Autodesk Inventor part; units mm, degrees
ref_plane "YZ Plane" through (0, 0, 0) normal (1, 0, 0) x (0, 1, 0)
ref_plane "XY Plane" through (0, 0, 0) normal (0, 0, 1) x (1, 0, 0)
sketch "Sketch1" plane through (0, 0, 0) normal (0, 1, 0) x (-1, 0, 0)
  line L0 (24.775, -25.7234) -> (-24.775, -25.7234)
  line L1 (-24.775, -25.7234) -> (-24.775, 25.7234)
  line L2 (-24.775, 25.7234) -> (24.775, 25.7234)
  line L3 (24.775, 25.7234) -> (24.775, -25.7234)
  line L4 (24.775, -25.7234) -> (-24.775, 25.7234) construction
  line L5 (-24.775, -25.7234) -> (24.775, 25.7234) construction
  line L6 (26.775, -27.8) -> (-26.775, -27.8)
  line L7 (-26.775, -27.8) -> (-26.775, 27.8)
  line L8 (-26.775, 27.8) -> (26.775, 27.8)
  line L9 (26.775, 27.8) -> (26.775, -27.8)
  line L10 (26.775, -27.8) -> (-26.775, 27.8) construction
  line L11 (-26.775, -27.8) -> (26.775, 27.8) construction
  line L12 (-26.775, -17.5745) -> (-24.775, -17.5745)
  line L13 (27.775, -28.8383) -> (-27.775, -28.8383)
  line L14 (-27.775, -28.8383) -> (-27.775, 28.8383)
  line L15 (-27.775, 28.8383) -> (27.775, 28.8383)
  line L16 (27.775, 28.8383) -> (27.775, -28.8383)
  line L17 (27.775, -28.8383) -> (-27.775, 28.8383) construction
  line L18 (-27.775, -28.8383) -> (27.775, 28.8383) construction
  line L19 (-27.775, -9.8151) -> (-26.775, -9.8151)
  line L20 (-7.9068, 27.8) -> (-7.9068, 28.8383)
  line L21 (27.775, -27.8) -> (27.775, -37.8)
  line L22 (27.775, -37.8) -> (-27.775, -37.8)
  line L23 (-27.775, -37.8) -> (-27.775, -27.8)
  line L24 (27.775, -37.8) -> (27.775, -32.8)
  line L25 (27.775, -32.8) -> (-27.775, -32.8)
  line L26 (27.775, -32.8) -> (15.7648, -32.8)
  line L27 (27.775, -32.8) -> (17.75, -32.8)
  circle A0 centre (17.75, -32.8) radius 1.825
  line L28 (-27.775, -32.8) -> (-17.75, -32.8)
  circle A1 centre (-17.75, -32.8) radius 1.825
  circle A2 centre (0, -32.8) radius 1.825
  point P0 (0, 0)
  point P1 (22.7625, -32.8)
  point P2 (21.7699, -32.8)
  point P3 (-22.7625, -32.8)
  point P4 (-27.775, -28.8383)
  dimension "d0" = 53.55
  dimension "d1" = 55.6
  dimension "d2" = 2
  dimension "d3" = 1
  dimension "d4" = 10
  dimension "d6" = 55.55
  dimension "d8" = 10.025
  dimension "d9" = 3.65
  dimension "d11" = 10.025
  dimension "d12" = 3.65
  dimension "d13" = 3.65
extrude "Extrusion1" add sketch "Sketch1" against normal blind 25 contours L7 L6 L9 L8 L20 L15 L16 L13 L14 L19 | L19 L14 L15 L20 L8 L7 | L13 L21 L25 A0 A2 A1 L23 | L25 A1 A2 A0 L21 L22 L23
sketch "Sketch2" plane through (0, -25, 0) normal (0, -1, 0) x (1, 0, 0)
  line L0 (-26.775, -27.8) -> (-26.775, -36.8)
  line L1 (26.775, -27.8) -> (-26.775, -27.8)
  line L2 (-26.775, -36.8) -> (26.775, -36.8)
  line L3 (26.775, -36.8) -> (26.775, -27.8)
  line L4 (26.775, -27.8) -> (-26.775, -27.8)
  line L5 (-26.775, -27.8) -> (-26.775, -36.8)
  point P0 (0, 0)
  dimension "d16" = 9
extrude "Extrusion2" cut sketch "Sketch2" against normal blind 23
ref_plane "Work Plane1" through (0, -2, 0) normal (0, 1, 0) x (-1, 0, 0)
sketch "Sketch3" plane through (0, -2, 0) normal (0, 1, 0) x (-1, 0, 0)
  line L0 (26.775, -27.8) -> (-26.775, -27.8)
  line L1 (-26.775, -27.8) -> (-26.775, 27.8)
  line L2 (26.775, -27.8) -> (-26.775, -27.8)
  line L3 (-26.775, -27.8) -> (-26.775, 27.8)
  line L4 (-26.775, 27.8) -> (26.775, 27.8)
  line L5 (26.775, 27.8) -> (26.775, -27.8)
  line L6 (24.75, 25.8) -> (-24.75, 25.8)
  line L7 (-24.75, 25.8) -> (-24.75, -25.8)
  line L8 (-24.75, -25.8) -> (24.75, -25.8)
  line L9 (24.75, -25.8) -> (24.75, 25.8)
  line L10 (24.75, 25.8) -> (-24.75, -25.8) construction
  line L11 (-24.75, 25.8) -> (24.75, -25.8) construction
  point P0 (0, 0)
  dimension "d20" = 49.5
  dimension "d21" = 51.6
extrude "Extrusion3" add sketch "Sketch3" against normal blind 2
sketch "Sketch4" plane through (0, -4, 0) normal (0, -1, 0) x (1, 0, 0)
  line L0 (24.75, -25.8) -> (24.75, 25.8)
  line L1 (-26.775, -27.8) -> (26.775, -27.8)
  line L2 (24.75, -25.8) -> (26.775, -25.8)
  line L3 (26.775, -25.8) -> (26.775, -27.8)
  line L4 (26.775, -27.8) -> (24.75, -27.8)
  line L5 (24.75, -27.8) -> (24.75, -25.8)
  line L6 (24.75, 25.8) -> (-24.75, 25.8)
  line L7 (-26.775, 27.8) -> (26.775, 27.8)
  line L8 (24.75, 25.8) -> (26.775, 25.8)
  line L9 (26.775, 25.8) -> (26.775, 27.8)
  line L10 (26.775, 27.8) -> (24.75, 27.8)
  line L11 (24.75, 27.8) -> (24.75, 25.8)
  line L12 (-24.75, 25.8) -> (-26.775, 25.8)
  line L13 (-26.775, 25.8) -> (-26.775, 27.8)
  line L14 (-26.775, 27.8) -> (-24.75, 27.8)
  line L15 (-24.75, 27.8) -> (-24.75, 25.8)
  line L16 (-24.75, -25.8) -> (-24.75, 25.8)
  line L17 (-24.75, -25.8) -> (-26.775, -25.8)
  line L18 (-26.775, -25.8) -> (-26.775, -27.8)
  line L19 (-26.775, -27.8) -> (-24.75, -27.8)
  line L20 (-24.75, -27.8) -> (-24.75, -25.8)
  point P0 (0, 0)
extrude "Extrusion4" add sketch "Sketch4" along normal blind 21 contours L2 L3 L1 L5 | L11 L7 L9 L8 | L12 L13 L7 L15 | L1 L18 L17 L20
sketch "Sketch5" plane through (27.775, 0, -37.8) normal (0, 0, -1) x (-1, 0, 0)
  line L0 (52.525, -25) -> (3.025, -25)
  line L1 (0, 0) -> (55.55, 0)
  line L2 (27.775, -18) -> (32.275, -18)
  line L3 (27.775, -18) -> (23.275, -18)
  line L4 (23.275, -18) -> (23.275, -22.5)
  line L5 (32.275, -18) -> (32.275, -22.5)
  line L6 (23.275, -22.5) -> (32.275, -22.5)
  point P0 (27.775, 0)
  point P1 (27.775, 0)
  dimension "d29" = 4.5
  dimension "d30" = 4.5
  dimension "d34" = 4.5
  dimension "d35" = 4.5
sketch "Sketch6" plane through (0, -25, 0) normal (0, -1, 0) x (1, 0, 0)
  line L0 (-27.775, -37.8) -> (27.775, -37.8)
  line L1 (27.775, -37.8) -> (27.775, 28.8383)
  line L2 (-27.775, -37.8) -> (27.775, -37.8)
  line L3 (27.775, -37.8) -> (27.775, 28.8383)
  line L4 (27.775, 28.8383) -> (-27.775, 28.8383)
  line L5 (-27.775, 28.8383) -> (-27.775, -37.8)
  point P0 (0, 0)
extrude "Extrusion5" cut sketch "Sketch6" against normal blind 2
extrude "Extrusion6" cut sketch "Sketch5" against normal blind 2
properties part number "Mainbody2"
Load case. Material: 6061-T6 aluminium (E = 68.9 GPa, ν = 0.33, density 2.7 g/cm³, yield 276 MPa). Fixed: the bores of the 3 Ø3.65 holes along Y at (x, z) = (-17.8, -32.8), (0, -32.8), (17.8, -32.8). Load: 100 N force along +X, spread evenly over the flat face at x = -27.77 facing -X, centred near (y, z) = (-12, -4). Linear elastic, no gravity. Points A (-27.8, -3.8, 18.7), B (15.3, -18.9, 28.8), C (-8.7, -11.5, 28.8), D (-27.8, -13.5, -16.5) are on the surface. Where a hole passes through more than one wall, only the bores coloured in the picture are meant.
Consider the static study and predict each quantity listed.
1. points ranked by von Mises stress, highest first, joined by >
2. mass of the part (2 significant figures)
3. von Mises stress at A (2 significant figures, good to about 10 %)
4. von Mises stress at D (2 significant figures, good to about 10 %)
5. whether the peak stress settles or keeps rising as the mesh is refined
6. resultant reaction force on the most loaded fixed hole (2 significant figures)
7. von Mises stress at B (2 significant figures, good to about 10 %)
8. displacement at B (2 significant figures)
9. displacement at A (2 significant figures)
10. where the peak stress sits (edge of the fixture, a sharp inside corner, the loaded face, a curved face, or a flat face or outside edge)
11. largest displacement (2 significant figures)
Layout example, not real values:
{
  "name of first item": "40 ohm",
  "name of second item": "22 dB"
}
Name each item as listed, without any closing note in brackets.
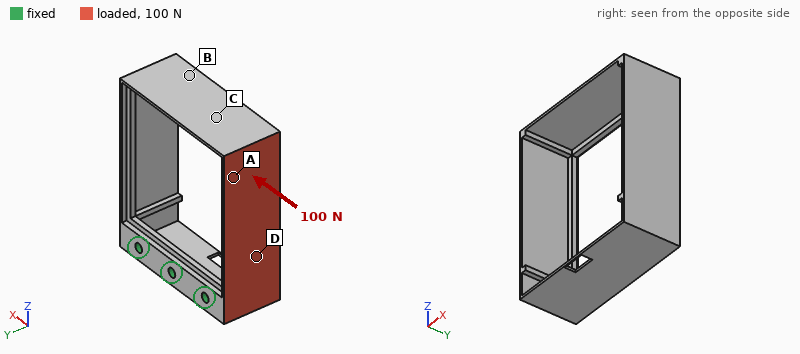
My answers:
{
  "points ranked by von Mises stress, highest first, joined by >": "A > D > B > C",
  "mass of the part": "20 g",
  "von Mises stress at A": "45 MPa",
  "von Mises stress at D": "29 MPa",
  "whether the peak stress settles or keeps rising as the mesh is refined": "keeps rising",
  "resultant reaction force on the most loaded fixed hole": "76 N",
  "von Mises stress at B": "16 MPa",
  "displacement at B": "0.73 mm",
  "displacement at A": "0.63 mm",
  "where the peak stress sits": "a sharp inside corner",
  "largest displacement": "0.80 mm"
}
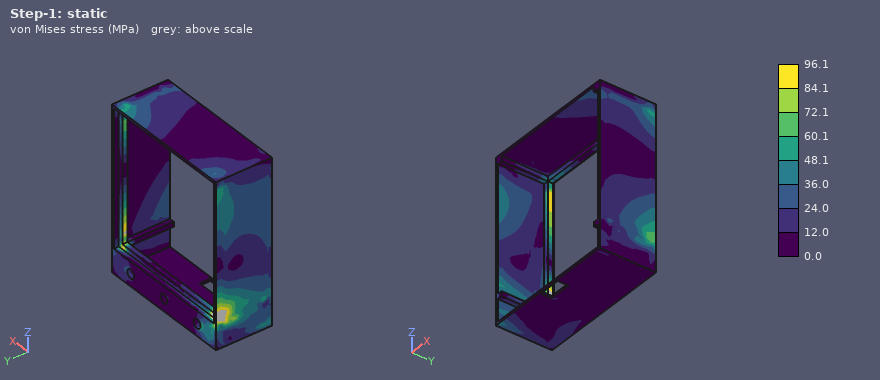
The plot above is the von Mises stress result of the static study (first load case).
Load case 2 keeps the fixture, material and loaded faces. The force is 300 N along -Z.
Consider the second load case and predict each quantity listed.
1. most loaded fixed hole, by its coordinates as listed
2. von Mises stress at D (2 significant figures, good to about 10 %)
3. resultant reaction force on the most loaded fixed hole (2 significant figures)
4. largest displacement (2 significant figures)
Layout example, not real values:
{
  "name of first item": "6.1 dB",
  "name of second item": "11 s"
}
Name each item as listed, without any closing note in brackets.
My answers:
{
  "most loaded fixed hole, by its coordinates as listed": "(-17.8, -32.8)",
  "von Mises stress at D": "20 MPa",
  "resultant reaction force on the most loaded fixed hole": "370 N",
  "largest displacement": "0.94 mm"
}
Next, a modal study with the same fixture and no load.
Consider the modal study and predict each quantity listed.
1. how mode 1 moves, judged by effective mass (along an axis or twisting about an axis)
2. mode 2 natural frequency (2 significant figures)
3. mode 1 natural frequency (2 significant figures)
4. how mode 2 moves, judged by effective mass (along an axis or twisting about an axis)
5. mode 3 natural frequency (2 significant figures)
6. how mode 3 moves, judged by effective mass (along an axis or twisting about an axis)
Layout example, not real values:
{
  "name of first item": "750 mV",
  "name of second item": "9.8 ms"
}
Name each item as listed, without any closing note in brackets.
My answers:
{
  "how mode 1 moves, judged by effective mass": "along X",
  "mode 2 natural frequency": "580 Hz",
  "mode 1 natural frequency": "460 Hz",
  "how mode 2 moves, judged by effective mass": "along Y",
  "mode 3 natural frequency": "760 Hz",
  "how mode 3 moves, judged by effective mass": "twisting about Z"
}
